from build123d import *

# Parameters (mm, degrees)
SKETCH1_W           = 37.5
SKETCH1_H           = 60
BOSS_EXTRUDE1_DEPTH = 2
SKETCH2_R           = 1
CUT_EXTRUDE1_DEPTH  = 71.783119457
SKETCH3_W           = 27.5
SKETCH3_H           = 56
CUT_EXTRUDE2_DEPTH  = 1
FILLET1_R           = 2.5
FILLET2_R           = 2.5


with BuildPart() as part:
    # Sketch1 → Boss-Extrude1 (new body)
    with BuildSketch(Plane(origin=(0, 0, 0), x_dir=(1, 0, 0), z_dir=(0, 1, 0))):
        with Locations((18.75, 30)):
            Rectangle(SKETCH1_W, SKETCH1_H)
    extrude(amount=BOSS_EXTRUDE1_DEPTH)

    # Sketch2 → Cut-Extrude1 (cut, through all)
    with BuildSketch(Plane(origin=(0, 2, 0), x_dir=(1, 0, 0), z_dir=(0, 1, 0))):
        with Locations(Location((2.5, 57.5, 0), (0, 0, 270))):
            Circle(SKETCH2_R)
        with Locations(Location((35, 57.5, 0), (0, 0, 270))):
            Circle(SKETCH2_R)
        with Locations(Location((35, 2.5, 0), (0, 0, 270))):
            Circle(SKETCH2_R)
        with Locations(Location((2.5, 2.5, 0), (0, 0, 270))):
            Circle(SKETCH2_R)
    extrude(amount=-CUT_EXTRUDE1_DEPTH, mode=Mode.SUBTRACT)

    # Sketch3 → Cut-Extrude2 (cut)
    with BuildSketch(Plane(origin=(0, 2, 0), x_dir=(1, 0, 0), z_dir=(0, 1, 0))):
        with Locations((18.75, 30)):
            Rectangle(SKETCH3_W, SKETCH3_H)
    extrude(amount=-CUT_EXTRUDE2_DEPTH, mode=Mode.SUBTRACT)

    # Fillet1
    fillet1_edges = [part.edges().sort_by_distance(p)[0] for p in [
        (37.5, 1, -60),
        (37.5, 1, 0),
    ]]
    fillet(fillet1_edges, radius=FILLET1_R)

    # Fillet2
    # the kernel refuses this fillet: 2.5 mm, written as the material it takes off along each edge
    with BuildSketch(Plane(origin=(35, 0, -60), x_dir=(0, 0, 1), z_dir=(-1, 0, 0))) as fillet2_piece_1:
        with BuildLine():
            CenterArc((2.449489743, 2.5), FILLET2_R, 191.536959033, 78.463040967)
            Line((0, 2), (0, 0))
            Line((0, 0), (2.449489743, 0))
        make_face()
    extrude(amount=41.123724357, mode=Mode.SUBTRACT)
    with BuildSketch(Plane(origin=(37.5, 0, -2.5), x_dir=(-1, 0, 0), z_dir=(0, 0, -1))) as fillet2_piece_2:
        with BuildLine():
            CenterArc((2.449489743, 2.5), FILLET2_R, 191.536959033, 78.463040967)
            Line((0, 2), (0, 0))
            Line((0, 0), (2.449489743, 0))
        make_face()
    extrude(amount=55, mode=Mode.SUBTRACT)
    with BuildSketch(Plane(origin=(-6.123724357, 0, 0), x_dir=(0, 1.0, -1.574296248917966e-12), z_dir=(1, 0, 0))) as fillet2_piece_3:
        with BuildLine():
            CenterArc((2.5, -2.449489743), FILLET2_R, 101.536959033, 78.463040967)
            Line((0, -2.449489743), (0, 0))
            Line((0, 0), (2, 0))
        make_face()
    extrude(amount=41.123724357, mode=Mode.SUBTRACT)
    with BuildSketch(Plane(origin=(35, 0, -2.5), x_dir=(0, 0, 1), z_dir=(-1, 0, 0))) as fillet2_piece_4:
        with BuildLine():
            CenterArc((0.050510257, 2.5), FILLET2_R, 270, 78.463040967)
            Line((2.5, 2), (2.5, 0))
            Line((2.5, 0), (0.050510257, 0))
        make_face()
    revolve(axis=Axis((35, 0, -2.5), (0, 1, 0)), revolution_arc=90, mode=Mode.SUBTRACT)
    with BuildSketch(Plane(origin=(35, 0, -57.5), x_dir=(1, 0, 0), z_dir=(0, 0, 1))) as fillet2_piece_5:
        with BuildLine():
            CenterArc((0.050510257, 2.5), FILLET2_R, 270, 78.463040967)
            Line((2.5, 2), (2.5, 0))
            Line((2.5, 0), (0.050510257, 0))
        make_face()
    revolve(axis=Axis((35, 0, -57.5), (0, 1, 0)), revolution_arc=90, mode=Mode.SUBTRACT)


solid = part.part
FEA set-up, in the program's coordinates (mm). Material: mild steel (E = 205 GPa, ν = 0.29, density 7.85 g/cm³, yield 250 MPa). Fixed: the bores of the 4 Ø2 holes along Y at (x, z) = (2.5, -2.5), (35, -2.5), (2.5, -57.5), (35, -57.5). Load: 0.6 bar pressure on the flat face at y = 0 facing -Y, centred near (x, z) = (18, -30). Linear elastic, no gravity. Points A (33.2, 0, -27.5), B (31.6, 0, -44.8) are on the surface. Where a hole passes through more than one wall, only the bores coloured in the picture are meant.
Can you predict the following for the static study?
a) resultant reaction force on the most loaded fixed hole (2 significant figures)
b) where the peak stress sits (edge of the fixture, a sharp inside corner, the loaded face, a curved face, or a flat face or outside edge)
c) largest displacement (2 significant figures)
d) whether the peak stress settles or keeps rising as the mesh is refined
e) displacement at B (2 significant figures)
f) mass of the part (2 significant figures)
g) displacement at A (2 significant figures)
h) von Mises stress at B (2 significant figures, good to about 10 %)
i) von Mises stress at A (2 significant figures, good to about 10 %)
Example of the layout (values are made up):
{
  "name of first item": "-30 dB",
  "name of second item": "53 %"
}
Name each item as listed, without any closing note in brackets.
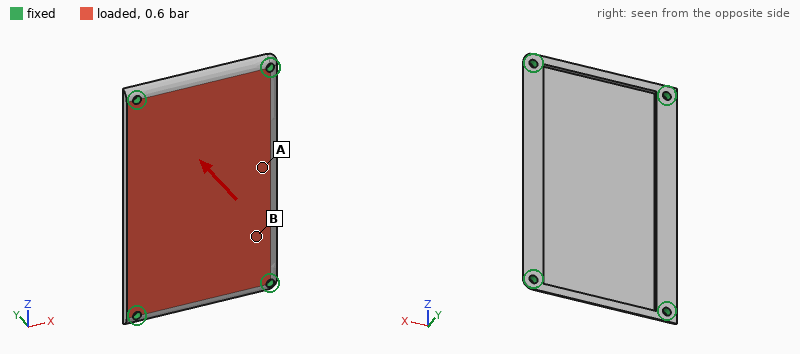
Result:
{
  "resultant reaction force on the most loaded fixed hole": "56 N",
  "where the peak stress sits": "edge of the fixture",
  "largest displacement": "37 µm",
  "whether the peak stress settles or keeps rising as the mesh is refined": "keeps rising",
  "displacement at B": "15 µm",
  "mass of the part": "22 g",
  "displacement at A": "25 µm",
  "von Mises stress at B": "8.1 MPa",
  "von Mises stress at A": "22 MPa"
}
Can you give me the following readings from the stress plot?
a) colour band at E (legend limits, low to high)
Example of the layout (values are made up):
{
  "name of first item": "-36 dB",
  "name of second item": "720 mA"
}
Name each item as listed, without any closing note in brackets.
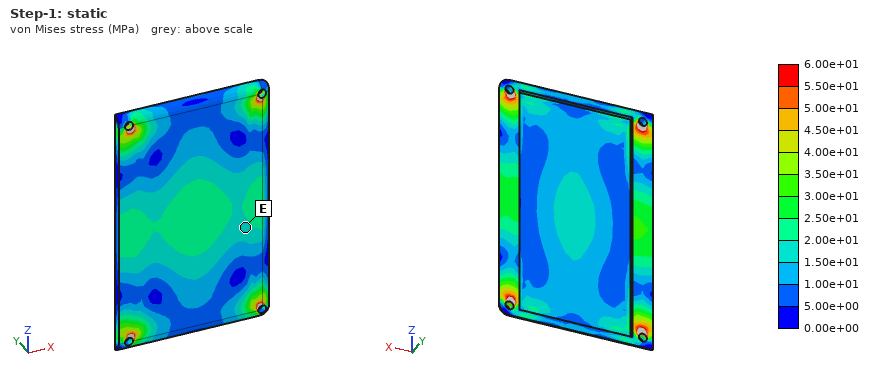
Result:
{
  "colour band at E": "1.50e+01 to 2.00e+01 MPa"
}
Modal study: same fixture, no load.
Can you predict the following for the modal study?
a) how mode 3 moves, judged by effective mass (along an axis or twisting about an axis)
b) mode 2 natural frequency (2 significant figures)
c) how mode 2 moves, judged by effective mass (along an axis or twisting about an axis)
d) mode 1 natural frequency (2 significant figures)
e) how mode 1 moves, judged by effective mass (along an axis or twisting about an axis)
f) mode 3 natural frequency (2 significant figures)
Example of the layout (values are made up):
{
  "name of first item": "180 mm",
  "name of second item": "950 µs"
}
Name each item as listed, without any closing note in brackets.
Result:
{
  "how mode 3 moves, judged by effective mass": "twisting about X",
  "mode 2 natural frequency": "3700 Hz",
  "how mode 2 moves, judged by effective mass": "twisting about Z",
  "mode 1 natural frequency": "2500 Hz",
  "how mode 1 moves, judged by effective mass": "along Y",
  "mode 3 natural frequency": "5900 Hz"
}
